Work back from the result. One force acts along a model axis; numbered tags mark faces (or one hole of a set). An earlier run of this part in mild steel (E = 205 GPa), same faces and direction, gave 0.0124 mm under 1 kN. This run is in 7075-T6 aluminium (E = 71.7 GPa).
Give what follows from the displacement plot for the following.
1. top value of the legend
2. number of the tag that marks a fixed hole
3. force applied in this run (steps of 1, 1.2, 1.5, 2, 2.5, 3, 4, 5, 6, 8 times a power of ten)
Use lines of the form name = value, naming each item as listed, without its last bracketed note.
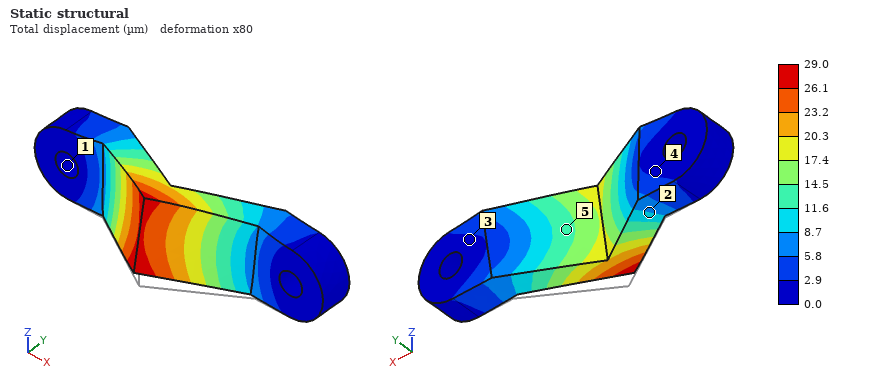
top value of the legend = 29.0 µm
number of the tag that marks a fixed hole = 1
force applied in this run = 800 N
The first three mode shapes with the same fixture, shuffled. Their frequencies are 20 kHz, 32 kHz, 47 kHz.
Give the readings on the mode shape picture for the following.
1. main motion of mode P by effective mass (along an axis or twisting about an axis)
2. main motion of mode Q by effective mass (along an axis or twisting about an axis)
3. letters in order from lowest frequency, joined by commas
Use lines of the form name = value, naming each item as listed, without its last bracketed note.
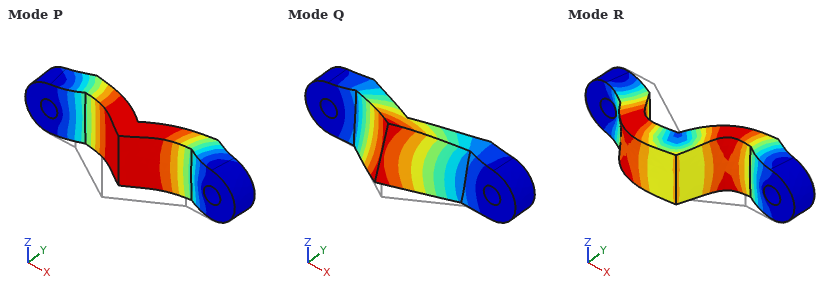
main motion of mode P by effective mass = along Y
main motion of mode Q by effective mass = along Z
letters in order from lowest frequency, joined by commas = Q, P, R
